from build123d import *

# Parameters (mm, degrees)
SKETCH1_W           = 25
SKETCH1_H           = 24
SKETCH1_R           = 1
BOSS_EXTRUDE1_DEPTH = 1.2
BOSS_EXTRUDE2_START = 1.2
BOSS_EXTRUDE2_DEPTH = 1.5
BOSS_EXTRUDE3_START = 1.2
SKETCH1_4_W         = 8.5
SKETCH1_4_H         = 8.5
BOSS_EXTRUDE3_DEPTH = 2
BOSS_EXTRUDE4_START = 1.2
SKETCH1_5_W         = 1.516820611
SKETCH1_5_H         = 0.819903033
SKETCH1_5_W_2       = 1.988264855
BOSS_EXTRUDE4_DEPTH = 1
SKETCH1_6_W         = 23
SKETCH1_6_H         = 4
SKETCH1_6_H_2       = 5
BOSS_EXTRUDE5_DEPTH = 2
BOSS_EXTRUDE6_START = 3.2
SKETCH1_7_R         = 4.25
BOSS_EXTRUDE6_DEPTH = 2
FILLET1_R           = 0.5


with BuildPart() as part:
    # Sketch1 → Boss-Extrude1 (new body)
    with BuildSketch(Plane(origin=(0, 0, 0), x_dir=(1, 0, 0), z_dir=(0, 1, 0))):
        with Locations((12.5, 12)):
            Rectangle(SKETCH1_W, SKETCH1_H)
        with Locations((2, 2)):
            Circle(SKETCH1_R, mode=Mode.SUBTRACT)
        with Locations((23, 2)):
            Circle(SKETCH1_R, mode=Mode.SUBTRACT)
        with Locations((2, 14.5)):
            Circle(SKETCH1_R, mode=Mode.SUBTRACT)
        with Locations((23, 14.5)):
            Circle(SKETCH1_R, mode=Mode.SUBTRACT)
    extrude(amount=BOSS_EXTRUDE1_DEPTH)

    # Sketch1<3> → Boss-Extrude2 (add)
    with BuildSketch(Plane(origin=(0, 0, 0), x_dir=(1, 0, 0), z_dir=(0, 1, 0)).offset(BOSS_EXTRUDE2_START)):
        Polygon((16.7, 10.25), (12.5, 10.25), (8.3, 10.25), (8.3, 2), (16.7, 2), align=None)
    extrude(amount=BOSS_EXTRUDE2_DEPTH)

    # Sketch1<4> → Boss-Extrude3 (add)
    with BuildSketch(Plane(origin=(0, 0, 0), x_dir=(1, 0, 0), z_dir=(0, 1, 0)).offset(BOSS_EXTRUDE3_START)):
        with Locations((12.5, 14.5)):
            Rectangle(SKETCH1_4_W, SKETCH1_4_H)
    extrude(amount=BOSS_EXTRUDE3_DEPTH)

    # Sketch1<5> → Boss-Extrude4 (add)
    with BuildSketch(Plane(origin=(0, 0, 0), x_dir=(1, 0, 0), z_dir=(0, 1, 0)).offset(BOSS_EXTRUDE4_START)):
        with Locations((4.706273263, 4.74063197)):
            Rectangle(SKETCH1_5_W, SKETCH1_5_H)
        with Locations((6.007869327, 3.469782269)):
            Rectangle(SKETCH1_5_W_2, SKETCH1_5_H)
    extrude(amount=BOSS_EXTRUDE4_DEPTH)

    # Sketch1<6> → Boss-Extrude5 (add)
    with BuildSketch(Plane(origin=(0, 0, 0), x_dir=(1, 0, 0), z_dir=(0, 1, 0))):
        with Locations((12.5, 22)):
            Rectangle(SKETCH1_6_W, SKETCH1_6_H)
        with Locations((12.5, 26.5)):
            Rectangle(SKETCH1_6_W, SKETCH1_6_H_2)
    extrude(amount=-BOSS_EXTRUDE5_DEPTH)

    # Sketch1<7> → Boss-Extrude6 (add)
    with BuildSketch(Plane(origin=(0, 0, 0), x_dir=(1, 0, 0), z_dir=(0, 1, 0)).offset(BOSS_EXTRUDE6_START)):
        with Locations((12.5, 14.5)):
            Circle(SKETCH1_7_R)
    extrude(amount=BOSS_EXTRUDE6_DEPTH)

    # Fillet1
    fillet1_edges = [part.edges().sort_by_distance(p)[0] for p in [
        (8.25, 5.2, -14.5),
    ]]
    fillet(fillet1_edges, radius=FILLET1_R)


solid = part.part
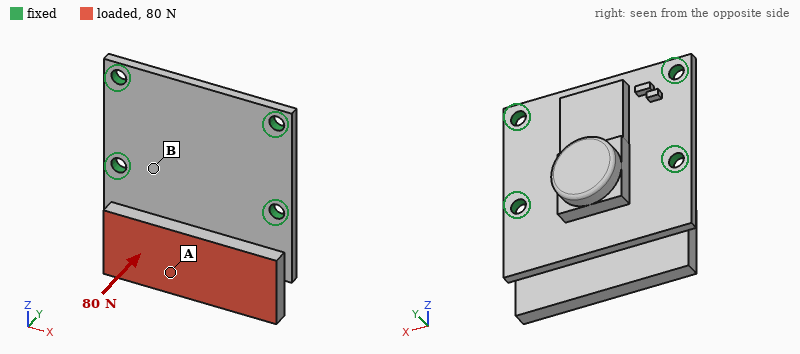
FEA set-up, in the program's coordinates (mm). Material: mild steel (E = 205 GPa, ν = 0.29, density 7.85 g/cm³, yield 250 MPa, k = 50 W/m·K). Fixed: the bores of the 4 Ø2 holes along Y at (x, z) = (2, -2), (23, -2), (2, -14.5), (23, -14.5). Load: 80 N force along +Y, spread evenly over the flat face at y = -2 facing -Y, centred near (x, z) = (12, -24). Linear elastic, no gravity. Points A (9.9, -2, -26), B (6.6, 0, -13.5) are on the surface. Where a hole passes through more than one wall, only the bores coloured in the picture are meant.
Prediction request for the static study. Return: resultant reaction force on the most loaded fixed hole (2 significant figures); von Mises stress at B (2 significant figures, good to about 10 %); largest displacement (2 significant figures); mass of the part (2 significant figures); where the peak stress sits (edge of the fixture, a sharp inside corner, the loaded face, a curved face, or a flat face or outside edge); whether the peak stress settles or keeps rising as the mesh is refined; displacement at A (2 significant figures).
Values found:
66 N
27 MPa
37 µm
12 g
edge of the fixture
keeps rising
28 µm
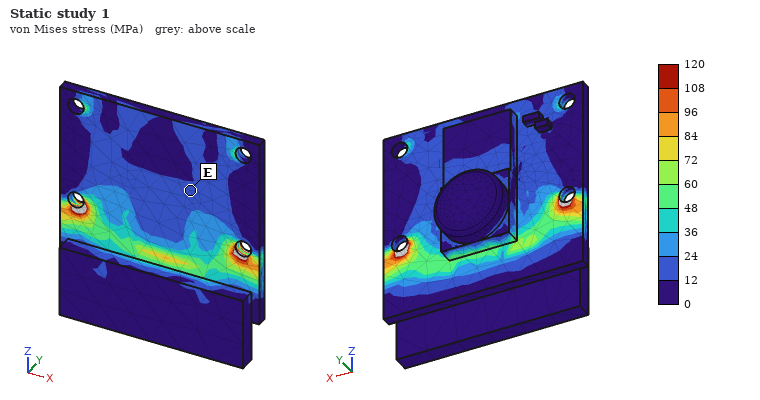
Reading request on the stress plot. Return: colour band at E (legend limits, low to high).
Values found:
12 to 24 MPa
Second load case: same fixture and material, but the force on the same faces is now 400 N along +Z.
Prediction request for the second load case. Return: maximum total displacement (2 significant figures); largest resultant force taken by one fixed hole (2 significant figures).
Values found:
65 µm
180 N
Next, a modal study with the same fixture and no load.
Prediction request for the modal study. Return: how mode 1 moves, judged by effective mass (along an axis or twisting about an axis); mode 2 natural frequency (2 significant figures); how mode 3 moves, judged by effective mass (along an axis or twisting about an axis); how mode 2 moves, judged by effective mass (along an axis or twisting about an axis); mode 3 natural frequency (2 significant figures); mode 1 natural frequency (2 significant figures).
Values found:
along Y
12 kHz
along Y
twisting about Z
14 kHz
4500 Hz
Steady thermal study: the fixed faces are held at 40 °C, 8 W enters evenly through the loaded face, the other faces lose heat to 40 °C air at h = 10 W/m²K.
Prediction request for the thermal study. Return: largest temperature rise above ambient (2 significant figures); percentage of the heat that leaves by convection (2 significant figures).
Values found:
51 K
4.1 %
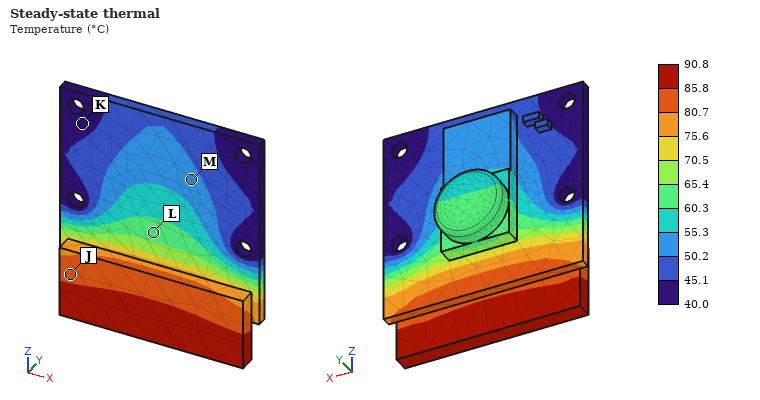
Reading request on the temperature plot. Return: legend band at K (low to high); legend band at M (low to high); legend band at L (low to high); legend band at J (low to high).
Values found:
40.0 to 45.1 °C
50.2 to 55.3 °C
60.3 to 65.4 °C
80.7 to 85.8 °C
